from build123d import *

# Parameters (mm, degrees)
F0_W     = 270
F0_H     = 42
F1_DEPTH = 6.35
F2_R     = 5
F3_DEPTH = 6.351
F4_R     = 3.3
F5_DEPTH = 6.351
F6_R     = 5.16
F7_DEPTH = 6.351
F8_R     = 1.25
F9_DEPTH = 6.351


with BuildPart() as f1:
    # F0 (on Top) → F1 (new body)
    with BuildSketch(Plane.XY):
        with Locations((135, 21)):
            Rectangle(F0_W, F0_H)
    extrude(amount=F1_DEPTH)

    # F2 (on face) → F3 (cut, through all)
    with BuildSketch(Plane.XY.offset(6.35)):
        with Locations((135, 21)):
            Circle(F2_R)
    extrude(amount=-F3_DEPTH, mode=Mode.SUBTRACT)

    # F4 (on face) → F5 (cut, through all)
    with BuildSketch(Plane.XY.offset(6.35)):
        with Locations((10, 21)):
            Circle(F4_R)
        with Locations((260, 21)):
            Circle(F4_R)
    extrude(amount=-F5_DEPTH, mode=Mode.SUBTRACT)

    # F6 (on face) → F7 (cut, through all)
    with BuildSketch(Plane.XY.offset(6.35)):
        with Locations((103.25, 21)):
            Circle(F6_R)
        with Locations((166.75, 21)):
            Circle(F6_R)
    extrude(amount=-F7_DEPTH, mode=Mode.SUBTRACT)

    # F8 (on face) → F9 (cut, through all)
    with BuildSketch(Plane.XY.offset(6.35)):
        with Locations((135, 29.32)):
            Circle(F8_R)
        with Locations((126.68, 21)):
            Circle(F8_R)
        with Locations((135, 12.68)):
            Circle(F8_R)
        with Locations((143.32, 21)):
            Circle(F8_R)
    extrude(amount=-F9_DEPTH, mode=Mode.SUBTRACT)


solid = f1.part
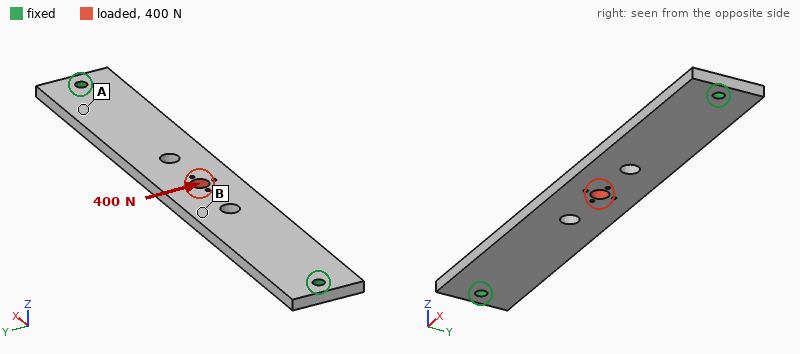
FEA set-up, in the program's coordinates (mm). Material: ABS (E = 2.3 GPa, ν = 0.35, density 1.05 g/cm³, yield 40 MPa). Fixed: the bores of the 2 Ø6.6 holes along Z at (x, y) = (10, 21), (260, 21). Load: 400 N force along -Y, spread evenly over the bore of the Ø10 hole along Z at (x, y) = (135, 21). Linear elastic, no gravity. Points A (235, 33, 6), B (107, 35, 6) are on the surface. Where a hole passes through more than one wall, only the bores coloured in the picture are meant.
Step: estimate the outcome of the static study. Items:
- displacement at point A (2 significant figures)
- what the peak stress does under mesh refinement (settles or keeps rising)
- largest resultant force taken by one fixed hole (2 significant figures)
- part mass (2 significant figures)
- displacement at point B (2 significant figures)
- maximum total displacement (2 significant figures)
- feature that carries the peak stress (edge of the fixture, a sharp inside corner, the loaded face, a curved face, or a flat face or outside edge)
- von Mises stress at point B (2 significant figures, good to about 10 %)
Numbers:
0.27 mm
keeps rising
200 N
73 g
0.92 mm
1.0 mm
edge of the fixture
5.2 MPa
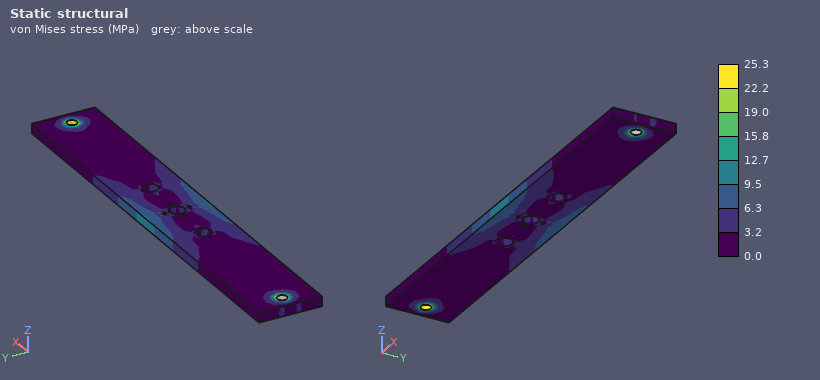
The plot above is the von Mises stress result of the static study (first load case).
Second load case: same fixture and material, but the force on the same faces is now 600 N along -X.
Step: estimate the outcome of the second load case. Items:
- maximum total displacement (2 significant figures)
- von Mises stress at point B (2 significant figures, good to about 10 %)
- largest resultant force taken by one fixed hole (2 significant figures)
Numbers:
85 µm
1.2 MPa
300 N
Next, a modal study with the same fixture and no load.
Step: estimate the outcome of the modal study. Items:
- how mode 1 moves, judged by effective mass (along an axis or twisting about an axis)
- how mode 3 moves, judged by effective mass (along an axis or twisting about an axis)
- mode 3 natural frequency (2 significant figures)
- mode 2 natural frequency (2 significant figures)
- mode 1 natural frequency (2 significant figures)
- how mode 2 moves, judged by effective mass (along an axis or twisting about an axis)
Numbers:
along Z
twisting about X
510 Hz
410 Hz
150 Hz
twisting about Y
